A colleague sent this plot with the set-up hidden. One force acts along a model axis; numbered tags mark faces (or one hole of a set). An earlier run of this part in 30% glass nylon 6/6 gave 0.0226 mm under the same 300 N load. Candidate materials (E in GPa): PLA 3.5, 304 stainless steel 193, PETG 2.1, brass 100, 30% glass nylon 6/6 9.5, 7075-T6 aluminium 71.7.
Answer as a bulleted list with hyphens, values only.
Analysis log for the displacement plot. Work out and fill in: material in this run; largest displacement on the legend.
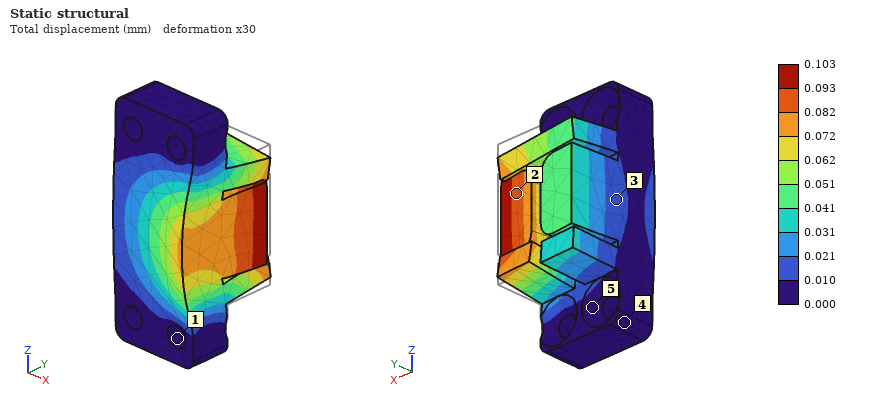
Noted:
- PETG
- 0.103 mm
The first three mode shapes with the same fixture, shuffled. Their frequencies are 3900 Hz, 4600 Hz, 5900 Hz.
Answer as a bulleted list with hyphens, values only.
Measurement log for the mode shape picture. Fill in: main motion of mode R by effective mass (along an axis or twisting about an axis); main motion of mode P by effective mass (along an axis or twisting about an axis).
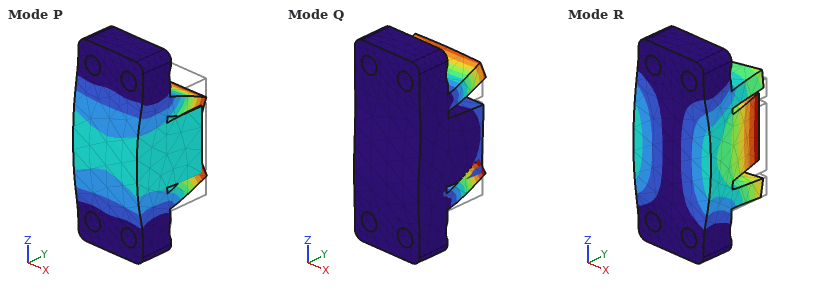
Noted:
- along X
- along Y
